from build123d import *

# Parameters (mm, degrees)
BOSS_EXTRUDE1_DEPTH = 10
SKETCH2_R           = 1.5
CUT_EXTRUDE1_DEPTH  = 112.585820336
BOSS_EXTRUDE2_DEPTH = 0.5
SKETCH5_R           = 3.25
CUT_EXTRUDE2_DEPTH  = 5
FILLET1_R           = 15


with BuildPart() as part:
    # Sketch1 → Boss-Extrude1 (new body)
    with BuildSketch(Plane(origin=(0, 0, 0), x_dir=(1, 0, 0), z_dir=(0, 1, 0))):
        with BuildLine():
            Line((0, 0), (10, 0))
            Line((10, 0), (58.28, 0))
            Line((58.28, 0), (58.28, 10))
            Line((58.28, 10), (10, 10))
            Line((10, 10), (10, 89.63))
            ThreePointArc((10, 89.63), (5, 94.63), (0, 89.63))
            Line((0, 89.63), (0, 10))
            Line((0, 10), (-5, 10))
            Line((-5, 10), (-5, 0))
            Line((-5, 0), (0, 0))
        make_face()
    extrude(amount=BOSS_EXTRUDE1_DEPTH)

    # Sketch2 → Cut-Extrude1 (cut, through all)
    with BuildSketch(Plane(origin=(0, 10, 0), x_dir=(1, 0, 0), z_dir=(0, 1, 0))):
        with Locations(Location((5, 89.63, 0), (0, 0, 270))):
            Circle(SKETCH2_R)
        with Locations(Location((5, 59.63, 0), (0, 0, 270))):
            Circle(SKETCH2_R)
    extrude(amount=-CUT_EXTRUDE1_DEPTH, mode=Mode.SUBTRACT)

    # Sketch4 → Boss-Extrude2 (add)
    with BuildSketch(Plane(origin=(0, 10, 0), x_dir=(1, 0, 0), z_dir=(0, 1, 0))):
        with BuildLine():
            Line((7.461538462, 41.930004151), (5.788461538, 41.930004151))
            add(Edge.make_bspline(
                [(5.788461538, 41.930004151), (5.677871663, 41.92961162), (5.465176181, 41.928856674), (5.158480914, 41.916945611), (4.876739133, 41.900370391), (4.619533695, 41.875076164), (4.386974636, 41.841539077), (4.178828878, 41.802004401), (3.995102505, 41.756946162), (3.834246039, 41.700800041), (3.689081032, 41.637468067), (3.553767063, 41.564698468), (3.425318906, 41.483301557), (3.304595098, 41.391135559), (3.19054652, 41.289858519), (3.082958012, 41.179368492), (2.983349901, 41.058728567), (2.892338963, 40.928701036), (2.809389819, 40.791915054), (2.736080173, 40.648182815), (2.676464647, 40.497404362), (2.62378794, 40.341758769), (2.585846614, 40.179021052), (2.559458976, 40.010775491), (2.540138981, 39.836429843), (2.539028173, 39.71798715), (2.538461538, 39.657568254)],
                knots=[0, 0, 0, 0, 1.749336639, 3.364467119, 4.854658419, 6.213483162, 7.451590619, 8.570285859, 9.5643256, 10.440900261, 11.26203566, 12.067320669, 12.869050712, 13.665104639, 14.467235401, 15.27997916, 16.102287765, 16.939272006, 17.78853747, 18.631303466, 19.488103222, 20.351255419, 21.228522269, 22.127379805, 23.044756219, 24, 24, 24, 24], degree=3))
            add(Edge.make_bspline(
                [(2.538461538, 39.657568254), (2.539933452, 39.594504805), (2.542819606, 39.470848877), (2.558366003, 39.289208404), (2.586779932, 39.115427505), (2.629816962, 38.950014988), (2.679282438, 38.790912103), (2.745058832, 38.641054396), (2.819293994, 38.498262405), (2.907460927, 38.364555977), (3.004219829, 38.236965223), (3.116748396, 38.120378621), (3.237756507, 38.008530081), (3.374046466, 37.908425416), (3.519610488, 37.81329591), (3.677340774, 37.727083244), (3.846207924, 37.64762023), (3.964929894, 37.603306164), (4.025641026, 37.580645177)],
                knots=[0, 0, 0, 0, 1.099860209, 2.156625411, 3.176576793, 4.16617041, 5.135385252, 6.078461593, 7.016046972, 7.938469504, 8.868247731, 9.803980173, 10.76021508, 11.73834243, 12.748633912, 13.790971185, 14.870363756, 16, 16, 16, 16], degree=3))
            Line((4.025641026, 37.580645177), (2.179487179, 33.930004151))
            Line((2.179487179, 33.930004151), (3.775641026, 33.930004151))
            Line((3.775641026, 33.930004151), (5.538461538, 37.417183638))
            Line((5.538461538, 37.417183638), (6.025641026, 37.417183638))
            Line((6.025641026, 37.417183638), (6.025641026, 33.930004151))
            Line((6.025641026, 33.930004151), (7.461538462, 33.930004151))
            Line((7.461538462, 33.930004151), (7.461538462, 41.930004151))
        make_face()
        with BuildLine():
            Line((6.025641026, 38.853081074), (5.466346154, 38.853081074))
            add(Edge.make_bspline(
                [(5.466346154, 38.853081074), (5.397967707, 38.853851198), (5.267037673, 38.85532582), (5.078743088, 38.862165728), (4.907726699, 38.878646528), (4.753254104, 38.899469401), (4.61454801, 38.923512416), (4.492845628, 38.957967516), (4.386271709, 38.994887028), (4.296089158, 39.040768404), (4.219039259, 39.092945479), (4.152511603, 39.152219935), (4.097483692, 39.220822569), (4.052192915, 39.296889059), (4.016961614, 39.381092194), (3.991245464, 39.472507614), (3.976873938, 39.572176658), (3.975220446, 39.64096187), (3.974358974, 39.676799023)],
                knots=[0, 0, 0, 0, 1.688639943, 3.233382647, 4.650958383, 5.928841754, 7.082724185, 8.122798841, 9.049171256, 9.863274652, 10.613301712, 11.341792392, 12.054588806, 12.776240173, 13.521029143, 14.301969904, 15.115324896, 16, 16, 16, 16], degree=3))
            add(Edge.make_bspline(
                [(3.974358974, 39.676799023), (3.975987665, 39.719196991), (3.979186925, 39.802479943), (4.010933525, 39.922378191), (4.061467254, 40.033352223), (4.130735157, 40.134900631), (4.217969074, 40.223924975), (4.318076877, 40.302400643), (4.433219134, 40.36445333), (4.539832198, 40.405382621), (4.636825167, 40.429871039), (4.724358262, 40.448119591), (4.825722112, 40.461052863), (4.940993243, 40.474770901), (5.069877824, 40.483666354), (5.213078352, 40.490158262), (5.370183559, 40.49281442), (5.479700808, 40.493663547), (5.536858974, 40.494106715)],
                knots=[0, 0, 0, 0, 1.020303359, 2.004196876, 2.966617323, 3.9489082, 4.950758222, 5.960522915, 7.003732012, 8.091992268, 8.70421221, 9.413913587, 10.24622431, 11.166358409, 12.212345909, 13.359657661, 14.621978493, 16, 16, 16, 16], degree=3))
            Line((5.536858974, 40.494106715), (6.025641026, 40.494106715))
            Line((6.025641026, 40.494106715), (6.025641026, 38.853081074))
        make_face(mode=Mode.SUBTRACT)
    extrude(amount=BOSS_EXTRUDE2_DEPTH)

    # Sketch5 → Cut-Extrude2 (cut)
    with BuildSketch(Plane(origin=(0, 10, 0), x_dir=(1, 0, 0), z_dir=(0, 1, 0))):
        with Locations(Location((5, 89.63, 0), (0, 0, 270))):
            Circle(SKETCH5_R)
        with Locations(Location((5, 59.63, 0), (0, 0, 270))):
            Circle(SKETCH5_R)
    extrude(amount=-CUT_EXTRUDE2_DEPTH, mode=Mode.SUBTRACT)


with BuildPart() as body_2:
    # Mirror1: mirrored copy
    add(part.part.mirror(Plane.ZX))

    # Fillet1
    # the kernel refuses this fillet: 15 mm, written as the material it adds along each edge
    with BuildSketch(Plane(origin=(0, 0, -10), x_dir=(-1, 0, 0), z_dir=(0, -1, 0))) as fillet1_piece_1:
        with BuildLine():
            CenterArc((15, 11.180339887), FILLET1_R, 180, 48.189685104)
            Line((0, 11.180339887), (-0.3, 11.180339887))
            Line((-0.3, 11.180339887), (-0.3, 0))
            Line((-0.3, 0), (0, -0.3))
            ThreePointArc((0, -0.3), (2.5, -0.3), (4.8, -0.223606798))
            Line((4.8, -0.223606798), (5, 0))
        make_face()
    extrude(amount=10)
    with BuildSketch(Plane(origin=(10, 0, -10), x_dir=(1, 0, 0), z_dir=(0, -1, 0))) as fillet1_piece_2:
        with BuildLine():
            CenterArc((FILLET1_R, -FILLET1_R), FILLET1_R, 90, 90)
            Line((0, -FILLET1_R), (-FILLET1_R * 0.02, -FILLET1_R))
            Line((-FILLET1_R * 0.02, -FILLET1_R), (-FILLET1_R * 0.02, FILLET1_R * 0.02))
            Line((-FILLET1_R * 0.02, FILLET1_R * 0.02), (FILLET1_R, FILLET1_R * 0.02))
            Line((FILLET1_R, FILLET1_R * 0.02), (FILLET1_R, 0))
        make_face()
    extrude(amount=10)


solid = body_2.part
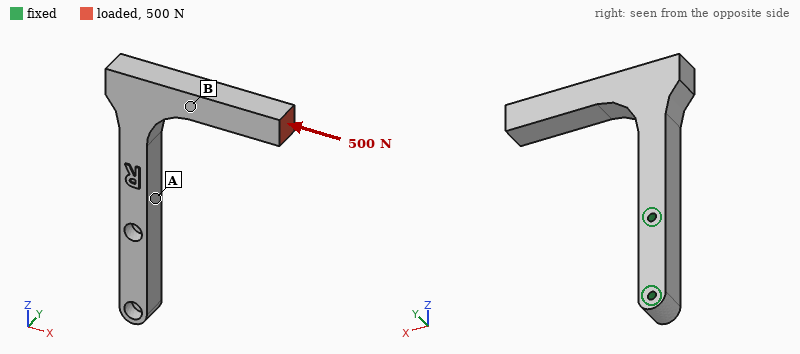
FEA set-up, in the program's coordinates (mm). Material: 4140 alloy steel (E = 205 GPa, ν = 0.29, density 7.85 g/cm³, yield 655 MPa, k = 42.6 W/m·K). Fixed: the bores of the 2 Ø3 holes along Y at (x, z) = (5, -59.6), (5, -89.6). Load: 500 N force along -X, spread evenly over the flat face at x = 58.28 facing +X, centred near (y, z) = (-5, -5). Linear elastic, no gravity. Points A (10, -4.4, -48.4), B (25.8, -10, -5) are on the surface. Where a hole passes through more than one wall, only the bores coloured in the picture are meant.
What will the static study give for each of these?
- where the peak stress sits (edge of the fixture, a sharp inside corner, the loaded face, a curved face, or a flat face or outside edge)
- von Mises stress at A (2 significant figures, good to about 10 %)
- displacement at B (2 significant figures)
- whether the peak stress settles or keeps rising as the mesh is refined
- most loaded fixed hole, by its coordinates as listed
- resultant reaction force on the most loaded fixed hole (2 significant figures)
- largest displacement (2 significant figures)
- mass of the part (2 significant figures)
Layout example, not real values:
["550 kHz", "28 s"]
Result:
["edge of the fixture", "130 MPa", "0.24 mm", "keeps rising", "(5, -59.6)", "1.1 kN", "0.37 mm", "120 g"]
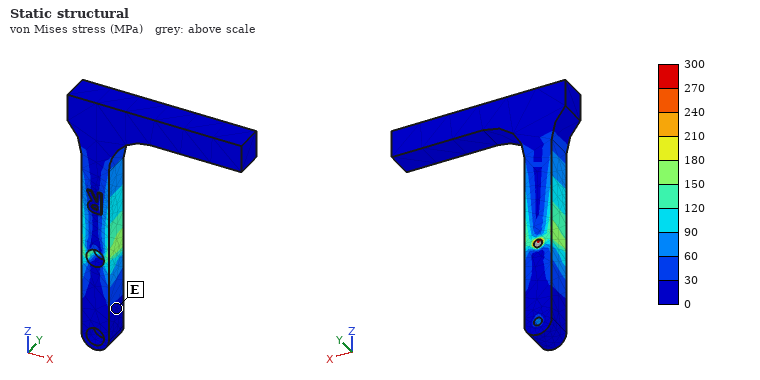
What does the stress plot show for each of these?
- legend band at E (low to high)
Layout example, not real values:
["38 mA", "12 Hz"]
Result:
["0 to 30 MPa"]
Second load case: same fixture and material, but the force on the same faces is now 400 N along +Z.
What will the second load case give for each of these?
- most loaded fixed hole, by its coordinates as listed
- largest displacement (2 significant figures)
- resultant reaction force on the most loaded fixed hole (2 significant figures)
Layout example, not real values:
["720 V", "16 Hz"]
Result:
["(5, -59.6)", "0.49 mm", "580 N"]
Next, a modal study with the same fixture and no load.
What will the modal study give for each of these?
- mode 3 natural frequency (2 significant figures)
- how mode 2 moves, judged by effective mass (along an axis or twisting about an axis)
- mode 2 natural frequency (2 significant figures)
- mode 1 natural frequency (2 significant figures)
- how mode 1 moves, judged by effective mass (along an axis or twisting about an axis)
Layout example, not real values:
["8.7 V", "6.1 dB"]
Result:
["1800 Hz", "along X", "820 Hz", "780 Hz", "along Y"]
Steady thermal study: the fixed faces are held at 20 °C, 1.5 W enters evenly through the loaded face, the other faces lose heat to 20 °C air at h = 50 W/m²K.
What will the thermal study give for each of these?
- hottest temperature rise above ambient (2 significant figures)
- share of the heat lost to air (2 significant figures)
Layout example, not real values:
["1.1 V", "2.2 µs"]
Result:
["15 K", "80 %"]
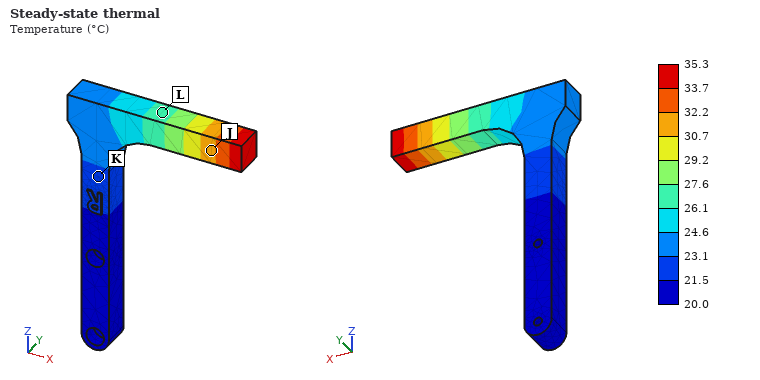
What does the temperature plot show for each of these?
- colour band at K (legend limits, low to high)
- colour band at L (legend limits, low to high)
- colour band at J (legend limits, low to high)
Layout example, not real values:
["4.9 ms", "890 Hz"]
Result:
["21.5 to 23.1 °C", "26.1 to 27.6 °C", "30.7 to 32.2 °C"]
